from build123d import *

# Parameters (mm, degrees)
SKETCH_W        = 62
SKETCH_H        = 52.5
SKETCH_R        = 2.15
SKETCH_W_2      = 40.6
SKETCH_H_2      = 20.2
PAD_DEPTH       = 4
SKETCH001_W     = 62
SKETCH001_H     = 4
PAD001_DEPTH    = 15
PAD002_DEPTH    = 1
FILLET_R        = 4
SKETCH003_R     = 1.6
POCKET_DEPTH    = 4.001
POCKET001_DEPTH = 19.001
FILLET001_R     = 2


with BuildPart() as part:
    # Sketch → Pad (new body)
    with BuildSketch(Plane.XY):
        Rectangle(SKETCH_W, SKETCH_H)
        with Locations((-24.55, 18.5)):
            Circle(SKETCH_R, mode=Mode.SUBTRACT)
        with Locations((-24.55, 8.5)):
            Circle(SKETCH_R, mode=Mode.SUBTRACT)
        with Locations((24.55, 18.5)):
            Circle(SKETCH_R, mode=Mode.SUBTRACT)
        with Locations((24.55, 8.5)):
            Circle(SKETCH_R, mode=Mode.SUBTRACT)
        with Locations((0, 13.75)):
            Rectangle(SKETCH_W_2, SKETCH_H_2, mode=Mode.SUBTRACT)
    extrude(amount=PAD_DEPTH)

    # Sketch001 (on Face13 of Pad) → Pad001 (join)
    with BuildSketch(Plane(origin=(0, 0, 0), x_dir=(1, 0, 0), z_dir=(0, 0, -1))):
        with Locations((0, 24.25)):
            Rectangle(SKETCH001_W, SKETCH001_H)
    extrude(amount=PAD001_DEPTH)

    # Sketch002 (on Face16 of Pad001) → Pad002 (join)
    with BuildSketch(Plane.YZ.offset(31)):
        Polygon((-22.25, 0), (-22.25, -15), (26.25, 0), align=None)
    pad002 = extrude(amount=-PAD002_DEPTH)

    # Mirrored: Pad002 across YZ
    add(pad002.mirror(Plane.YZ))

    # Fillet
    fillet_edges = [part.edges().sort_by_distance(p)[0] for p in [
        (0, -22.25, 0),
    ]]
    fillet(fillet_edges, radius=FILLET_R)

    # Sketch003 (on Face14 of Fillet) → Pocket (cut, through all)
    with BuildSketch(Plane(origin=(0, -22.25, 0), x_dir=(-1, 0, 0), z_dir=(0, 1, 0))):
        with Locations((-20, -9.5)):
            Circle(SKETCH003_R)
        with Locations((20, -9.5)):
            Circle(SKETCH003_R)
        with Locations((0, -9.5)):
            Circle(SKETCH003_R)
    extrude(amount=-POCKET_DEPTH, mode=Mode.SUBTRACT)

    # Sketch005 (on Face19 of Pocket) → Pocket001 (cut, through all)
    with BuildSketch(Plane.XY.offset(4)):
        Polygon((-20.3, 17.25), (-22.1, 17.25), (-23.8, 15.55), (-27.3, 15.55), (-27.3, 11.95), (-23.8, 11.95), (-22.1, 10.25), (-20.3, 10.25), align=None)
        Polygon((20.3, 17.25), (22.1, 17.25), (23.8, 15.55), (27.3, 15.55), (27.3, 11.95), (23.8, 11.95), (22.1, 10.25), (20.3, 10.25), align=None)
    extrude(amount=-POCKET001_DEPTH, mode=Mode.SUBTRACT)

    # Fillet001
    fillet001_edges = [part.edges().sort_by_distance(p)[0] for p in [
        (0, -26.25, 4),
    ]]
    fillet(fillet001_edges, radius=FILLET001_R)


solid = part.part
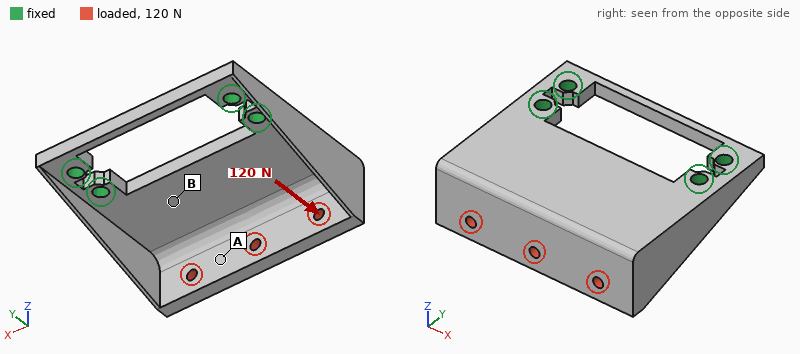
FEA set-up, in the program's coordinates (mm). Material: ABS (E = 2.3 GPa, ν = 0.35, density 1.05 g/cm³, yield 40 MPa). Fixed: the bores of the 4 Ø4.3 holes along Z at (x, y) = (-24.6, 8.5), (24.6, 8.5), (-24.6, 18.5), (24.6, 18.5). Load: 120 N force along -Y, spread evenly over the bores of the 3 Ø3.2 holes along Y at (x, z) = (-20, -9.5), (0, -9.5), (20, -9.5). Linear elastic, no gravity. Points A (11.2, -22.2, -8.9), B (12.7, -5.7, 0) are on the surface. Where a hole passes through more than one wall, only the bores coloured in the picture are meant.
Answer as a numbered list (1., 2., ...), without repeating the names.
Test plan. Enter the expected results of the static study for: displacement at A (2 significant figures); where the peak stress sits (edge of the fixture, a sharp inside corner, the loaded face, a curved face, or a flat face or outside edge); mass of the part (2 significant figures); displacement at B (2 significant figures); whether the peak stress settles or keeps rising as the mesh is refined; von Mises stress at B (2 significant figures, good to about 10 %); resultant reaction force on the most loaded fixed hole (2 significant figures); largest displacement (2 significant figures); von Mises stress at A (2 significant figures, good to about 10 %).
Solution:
1. 0.70 mm
2. edge of the fixture
3. 14 g
4. 0.15 mm
5. keeps rising
6. 3.0 MPa
7. 49 N
8. 0.98 mm
9. 1.6 MPa
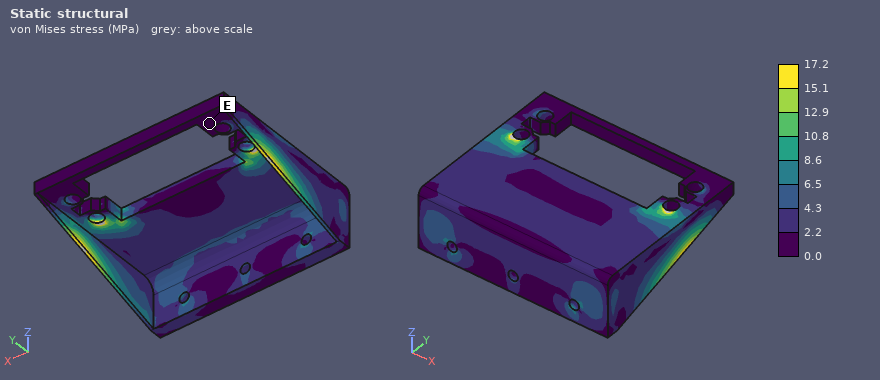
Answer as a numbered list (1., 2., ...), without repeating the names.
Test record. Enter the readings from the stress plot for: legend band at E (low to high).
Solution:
1. 0.0 to 2.2 MPa
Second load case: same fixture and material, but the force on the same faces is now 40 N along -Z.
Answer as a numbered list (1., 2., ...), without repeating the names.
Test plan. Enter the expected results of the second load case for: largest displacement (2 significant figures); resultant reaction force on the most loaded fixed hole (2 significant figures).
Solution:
1. 0.66 mm
2. 46 N
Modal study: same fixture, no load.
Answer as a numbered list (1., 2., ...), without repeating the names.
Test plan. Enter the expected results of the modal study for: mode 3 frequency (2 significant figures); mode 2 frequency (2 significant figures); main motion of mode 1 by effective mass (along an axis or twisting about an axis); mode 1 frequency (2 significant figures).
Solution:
1. 1900 Hz
2. 980 Hz
3. along Z
4. 510 Hz
